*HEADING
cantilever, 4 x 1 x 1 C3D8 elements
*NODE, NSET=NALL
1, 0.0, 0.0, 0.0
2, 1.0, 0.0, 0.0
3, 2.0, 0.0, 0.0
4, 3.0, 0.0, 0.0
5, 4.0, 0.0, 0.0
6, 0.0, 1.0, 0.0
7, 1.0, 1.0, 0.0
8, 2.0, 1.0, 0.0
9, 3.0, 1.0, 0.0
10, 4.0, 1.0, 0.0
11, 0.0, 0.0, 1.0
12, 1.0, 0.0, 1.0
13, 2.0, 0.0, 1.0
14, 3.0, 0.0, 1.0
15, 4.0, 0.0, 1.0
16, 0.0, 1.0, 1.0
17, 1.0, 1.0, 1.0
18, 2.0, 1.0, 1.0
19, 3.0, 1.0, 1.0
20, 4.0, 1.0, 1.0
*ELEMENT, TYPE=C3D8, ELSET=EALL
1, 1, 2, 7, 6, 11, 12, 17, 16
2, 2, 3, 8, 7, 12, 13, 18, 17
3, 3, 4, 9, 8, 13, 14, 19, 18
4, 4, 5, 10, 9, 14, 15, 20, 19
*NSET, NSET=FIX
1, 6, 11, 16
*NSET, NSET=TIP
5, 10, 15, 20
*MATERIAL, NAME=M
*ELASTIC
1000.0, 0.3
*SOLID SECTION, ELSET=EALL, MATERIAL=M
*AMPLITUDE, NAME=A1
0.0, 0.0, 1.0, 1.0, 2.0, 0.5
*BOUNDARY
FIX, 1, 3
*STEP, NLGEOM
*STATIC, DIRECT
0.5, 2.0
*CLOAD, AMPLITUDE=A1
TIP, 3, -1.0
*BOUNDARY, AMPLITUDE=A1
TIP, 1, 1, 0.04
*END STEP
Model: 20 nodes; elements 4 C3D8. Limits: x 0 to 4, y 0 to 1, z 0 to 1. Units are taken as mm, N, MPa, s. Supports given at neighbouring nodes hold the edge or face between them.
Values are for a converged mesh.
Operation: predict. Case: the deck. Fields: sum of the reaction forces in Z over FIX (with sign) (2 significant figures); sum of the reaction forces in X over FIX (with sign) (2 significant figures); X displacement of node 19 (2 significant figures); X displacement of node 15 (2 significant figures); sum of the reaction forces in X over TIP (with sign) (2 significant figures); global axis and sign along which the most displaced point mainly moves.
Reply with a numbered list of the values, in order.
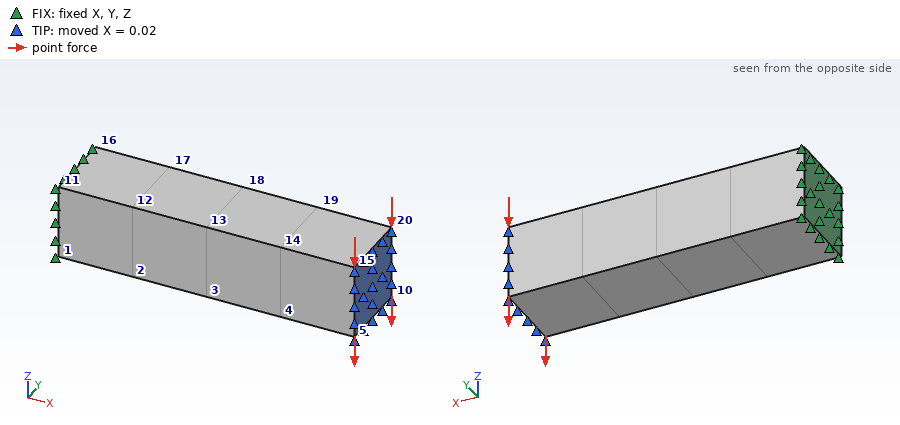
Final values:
1. 2.0 N
2. -5.7 N
3. 0.031 mm
4. 0.020 mm
5. 5.7 N
6. -Z
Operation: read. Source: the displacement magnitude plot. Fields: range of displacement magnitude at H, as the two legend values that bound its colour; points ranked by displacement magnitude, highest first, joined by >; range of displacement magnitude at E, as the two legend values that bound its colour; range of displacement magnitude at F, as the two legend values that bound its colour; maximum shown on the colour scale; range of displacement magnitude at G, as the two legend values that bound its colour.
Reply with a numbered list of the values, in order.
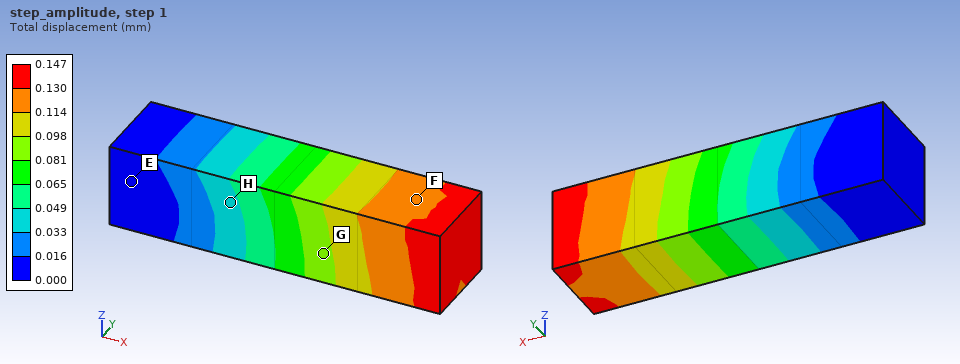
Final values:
1. 0.033 to 0.049 mm
2. F > G > H > E
3. 0.000 to 0.016 mm
4. 0.114 to 0.130 mm
5. 0.147 mm
6. 0.081 to 0.098 mm
